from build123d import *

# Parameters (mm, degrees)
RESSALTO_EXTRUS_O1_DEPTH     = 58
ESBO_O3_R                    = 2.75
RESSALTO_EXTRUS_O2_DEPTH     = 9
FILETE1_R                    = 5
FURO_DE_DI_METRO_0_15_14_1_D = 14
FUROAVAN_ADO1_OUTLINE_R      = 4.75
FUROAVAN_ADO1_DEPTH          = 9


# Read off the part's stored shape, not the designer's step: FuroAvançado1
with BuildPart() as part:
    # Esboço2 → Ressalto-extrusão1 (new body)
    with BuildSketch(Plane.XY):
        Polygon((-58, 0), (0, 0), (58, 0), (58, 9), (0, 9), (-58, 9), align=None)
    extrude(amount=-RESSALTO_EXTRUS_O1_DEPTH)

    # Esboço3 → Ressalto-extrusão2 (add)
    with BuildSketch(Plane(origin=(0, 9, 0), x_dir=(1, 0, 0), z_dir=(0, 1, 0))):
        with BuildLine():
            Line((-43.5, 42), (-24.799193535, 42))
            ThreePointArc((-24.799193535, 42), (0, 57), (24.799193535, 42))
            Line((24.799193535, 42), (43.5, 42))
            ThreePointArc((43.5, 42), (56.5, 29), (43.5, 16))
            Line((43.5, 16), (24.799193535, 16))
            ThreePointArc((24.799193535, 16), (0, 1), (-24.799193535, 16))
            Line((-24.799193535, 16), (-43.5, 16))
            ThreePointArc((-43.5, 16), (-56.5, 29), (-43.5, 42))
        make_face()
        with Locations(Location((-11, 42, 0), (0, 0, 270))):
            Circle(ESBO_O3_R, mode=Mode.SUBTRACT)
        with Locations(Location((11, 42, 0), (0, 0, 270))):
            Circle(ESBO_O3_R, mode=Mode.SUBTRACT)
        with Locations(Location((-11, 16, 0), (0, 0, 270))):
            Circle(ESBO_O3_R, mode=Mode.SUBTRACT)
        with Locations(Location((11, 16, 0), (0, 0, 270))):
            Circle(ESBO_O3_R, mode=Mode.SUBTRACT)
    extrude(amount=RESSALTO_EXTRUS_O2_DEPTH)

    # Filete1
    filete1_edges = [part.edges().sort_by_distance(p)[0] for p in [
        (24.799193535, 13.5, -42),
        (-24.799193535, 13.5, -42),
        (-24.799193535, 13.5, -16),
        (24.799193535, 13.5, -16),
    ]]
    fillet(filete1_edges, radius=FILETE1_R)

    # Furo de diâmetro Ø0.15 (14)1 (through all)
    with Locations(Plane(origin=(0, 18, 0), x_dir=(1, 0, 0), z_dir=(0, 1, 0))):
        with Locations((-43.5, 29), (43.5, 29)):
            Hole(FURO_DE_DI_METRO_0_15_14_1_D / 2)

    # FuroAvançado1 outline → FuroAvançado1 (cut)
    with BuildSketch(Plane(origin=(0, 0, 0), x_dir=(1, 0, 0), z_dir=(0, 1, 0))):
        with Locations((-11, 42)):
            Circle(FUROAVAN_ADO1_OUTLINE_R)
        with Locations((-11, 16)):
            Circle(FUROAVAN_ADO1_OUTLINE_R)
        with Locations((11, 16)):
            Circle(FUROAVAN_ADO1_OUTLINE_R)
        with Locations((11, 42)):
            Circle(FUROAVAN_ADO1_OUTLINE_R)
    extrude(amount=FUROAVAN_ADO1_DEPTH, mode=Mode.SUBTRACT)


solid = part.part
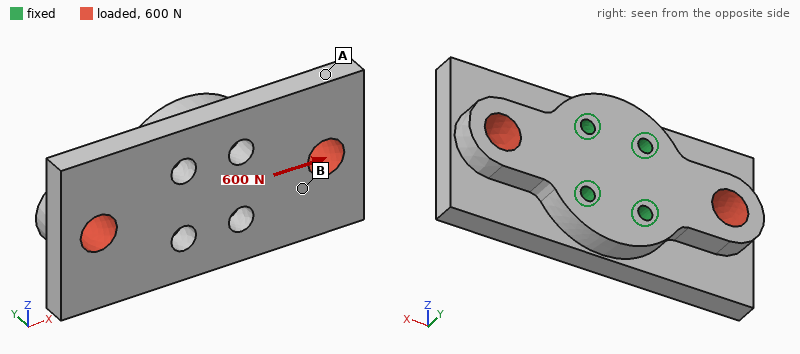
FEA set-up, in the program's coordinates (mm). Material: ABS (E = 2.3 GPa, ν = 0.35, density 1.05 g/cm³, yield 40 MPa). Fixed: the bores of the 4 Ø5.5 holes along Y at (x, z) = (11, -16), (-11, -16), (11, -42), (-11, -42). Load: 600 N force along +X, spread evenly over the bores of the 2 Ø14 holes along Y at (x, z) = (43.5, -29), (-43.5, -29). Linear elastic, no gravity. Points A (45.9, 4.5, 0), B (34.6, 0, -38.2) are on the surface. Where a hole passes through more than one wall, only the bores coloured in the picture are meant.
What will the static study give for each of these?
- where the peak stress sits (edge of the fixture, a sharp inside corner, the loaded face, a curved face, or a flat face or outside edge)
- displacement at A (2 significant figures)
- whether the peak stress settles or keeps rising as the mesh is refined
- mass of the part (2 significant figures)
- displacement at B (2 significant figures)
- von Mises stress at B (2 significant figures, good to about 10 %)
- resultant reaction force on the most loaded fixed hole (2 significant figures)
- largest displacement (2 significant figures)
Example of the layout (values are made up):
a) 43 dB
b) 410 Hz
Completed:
a) edge of the fixture
b) 12 µm
c) keeps rising
d) 91 g
e) 12 µm
f) 0.50 MPa
g) 160 N
h) 20 µm
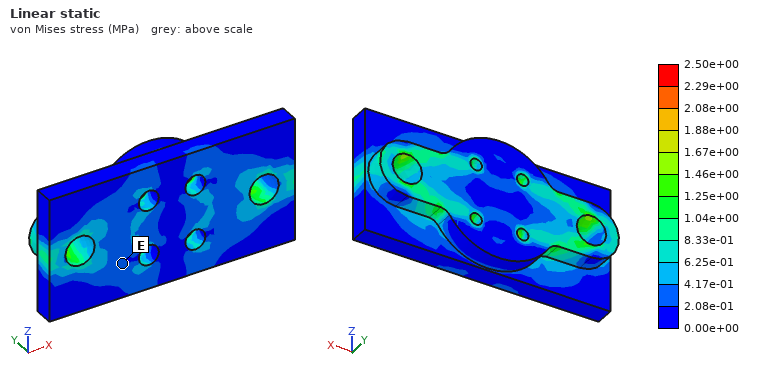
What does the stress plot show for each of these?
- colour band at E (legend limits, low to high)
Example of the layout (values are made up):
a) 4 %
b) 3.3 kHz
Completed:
a) 2.08e-01 to 4.17e-01 MPa
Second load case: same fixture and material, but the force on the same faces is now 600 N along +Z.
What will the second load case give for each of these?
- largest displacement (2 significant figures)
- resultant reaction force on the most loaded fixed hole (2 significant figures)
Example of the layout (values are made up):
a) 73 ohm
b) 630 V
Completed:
a) 50 µm
b) 180 N
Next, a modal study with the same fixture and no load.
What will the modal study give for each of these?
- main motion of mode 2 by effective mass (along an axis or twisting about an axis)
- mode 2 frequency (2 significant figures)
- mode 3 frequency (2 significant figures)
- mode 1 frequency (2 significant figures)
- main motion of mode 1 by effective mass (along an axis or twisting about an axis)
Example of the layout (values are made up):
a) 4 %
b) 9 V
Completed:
a) along Y
b) 1600 Hz
c) 2400 Hz
d) 1400 Hz
e) twisting about Z
